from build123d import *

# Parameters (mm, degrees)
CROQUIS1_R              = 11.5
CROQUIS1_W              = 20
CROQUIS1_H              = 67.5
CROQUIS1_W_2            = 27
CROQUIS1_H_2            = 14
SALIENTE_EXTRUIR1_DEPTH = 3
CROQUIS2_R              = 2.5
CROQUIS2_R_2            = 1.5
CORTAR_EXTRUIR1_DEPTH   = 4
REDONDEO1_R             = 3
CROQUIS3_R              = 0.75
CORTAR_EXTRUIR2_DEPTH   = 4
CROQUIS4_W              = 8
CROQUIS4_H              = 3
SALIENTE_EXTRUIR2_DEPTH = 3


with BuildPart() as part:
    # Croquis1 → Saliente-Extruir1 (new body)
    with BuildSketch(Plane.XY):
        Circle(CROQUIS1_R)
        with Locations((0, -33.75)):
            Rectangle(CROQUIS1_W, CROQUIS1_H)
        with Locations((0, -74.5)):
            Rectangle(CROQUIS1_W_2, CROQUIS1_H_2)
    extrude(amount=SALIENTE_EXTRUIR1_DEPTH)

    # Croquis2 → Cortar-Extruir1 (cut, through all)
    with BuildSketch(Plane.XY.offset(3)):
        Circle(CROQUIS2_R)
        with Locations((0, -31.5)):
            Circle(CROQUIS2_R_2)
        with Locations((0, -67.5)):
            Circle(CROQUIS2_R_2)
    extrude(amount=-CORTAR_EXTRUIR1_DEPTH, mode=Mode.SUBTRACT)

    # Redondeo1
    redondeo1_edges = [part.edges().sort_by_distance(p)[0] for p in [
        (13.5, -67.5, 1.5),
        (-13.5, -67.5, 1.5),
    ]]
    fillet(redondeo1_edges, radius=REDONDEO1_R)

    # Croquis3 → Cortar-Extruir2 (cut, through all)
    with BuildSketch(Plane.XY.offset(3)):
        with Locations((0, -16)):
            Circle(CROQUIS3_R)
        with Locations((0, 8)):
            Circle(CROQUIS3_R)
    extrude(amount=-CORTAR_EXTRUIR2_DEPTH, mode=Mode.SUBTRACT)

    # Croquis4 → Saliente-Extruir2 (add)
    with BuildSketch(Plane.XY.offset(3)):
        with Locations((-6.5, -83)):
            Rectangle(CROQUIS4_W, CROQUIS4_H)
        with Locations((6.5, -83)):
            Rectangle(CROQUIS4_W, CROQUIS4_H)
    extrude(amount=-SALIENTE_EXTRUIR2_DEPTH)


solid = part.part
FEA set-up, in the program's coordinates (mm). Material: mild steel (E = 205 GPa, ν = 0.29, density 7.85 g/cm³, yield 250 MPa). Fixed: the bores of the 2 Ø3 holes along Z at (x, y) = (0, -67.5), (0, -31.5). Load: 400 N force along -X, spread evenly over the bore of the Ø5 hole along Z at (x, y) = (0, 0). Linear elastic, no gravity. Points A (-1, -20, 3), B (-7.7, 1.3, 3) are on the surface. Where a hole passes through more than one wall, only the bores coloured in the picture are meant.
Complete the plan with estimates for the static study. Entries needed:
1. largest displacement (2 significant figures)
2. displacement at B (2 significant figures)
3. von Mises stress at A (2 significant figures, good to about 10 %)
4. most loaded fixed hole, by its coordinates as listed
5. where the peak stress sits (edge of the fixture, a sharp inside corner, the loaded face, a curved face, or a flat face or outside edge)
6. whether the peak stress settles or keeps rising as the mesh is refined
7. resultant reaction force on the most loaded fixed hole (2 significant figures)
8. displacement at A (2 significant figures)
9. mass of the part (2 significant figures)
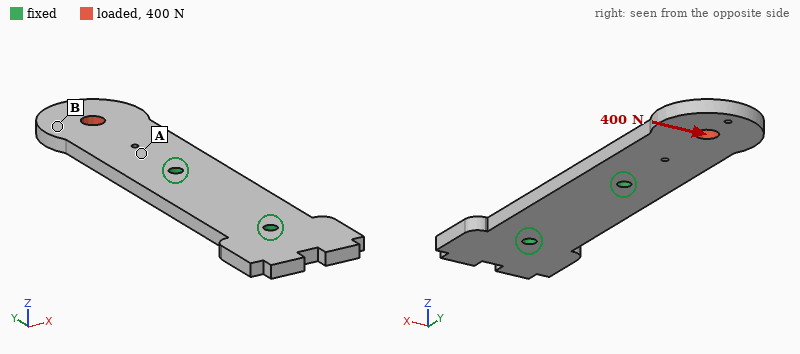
35 µm
27 µm
18 MPa
(0, -31.5)
edge of the fixture
keeps rising
690 N
7.1 µm
46 g
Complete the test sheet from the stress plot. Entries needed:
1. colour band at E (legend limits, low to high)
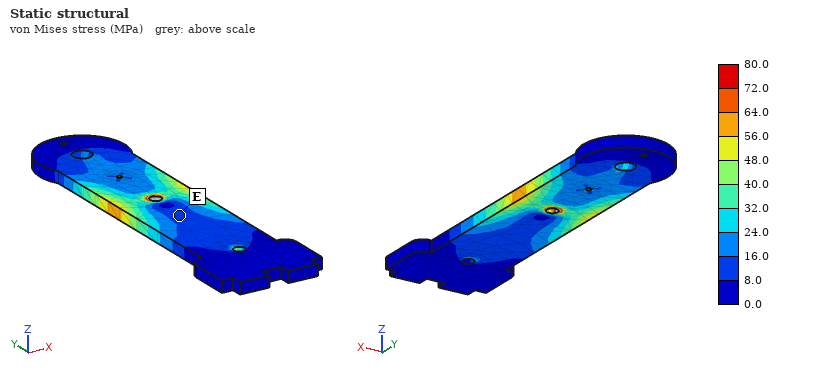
8.0 to 16.0 MPa
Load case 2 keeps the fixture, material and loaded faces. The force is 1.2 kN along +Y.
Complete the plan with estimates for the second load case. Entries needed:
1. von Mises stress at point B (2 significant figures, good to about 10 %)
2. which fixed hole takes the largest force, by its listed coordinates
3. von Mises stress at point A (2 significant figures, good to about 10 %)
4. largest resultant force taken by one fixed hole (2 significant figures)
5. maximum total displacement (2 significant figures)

8.5 MPa
(0, -31.5)
22 MPa
1.0 kN
4.5 µm
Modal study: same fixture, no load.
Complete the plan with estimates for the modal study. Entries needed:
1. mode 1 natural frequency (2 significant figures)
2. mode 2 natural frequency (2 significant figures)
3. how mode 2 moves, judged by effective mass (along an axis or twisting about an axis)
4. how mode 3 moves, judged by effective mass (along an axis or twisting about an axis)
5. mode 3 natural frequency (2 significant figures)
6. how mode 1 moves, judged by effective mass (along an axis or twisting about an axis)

1400 Hz
5200 Hz
twisting about Y
along X
5900 Hz
along Z
